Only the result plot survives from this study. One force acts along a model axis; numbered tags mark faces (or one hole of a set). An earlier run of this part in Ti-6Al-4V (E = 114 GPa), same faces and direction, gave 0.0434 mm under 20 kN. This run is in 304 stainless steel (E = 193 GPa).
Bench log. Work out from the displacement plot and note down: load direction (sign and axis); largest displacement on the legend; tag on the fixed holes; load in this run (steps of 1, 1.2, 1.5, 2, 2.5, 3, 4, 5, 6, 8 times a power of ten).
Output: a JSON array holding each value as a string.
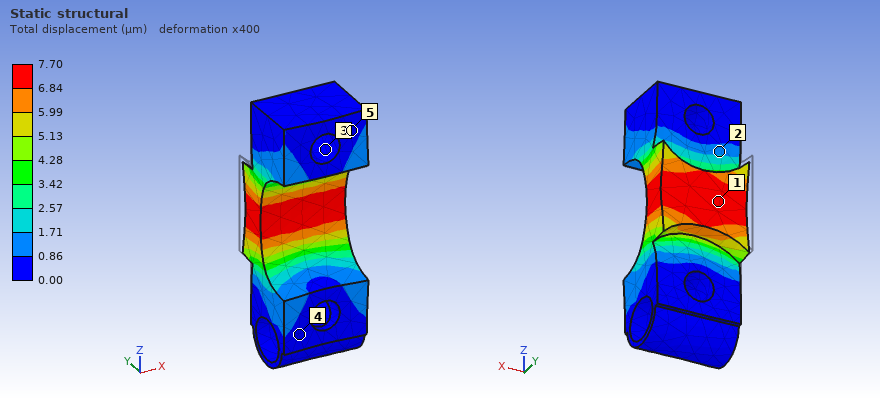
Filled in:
["-Y", "7.70 µm", "3", "6 kN"]
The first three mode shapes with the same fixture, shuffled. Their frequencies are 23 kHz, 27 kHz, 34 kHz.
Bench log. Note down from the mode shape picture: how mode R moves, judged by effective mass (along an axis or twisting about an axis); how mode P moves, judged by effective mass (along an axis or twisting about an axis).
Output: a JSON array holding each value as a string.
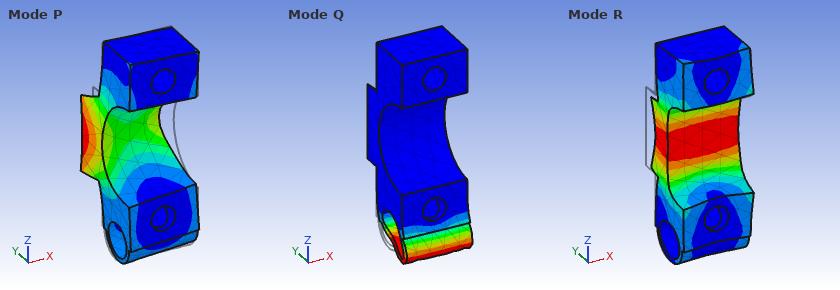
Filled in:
["along Y", "along X"]
